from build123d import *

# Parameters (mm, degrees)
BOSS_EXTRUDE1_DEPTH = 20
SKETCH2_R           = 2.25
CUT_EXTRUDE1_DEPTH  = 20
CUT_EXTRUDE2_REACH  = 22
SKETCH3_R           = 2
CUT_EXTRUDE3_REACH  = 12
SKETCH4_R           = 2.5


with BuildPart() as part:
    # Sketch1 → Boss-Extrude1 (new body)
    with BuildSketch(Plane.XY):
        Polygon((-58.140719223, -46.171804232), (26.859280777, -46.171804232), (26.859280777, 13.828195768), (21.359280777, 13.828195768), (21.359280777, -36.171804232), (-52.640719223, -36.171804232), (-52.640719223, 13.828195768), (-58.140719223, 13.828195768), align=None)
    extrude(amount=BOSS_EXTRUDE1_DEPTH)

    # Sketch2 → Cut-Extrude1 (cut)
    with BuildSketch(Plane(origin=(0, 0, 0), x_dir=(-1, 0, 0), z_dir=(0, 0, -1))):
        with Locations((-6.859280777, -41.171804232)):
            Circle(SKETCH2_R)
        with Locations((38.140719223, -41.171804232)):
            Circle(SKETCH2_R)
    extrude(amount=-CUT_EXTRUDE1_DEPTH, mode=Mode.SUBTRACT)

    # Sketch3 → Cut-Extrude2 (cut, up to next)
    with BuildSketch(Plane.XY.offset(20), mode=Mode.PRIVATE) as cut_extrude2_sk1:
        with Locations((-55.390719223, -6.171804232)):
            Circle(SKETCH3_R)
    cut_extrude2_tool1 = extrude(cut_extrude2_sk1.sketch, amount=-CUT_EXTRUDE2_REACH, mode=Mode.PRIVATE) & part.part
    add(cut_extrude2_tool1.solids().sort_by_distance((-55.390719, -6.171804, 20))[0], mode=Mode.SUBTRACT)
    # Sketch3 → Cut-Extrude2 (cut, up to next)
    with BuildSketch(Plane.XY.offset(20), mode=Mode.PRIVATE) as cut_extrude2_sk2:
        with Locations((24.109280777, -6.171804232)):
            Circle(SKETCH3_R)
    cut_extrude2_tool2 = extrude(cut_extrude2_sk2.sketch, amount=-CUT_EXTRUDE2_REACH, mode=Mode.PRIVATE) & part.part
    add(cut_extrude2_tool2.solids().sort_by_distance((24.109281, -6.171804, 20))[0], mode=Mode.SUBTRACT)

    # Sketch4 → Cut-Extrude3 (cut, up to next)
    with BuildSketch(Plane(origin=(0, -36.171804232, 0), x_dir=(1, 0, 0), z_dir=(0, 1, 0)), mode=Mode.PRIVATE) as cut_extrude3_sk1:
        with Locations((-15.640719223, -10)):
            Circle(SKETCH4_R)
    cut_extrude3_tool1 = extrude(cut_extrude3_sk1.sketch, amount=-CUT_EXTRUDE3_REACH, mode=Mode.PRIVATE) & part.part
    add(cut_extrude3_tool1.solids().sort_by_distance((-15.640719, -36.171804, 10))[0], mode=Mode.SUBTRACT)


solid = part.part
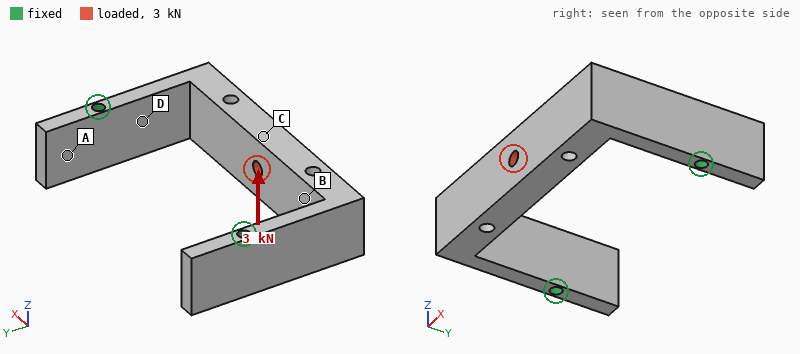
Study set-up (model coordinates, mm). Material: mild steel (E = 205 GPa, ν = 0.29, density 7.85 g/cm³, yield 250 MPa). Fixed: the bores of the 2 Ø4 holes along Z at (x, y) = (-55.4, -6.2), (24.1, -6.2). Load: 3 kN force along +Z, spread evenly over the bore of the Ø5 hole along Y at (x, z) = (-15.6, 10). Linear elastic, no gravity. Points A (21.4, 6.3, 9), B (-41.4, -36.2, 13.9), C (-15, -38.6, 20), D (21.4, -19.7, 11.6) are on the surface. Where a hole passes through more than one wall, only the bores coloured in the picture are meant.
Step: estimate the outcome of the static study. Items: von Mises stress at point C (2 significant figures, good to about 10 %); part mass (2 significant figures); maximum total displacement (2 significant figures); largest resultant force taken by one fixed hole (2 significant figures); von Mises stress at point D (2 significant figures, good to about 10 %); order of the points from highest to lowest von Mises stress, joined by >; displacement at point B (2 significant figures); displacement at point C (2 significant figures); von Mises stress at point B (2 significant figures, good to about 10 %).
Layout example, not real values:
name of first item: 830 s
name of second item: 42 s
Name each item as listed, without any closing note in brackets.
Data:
von Mises stress at point C: 87 MPa
part mass: 210 g
maximum total displacement: 65 µm
largest resultant force taken by one fixed hole: 1.5 kN
von Mises stress at point D: 63 MPa
order of the points from highest to lowest von Mises stress, joined by >: C > D > B > A
displacement at point B: 39 µm
displacement at point C: 56 µm
von Mises stress at point B: 31 MPa
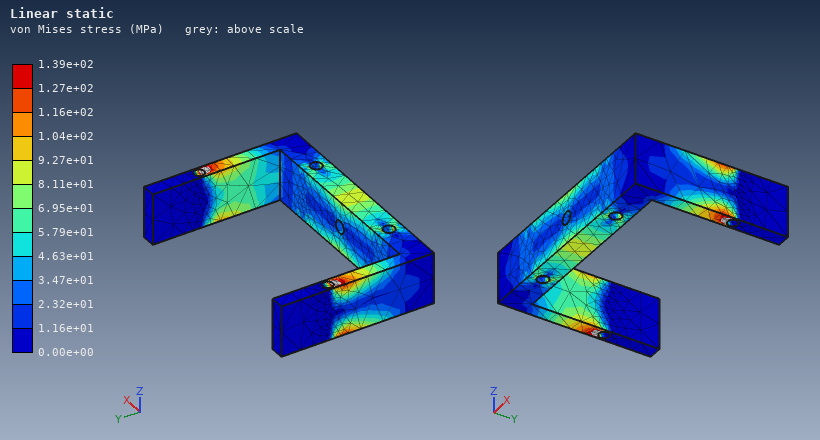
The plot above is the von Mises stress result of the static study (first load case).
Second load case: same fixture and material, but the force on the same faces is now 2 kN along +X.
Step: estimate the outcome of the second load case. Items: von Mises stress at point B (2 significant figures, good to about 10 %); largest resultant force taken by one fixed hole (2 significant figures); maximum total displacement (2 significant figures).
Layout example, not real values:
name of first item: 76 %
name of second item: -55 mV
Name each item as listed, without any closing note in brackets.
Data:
von Mises stress at point B: 45 MPa
largest resultant force taken by one fixed hole: 1.1 kN
maximum total displacement: 62 µm
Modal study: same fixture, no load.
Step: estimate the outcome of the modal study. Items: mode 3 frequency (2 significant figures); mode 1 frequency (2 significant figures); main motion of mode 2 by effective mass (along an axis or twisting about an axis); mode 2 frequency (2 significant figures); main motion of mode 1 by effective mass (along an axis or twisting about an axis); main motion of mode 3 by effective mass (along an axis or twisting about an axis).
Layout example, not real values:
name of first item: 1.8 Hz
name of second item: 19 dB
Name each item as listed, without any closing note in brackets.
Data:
mode 3 frequency: 4500 Hz
mode 1 frequency: 2500 Hz
main motion of mode 2 by effective mass: along Z
mode 2 frequency: 3700 Hz
main motion of mode 1 by effective mass: along X
main motion of mode 3 by effective mass: along Y
